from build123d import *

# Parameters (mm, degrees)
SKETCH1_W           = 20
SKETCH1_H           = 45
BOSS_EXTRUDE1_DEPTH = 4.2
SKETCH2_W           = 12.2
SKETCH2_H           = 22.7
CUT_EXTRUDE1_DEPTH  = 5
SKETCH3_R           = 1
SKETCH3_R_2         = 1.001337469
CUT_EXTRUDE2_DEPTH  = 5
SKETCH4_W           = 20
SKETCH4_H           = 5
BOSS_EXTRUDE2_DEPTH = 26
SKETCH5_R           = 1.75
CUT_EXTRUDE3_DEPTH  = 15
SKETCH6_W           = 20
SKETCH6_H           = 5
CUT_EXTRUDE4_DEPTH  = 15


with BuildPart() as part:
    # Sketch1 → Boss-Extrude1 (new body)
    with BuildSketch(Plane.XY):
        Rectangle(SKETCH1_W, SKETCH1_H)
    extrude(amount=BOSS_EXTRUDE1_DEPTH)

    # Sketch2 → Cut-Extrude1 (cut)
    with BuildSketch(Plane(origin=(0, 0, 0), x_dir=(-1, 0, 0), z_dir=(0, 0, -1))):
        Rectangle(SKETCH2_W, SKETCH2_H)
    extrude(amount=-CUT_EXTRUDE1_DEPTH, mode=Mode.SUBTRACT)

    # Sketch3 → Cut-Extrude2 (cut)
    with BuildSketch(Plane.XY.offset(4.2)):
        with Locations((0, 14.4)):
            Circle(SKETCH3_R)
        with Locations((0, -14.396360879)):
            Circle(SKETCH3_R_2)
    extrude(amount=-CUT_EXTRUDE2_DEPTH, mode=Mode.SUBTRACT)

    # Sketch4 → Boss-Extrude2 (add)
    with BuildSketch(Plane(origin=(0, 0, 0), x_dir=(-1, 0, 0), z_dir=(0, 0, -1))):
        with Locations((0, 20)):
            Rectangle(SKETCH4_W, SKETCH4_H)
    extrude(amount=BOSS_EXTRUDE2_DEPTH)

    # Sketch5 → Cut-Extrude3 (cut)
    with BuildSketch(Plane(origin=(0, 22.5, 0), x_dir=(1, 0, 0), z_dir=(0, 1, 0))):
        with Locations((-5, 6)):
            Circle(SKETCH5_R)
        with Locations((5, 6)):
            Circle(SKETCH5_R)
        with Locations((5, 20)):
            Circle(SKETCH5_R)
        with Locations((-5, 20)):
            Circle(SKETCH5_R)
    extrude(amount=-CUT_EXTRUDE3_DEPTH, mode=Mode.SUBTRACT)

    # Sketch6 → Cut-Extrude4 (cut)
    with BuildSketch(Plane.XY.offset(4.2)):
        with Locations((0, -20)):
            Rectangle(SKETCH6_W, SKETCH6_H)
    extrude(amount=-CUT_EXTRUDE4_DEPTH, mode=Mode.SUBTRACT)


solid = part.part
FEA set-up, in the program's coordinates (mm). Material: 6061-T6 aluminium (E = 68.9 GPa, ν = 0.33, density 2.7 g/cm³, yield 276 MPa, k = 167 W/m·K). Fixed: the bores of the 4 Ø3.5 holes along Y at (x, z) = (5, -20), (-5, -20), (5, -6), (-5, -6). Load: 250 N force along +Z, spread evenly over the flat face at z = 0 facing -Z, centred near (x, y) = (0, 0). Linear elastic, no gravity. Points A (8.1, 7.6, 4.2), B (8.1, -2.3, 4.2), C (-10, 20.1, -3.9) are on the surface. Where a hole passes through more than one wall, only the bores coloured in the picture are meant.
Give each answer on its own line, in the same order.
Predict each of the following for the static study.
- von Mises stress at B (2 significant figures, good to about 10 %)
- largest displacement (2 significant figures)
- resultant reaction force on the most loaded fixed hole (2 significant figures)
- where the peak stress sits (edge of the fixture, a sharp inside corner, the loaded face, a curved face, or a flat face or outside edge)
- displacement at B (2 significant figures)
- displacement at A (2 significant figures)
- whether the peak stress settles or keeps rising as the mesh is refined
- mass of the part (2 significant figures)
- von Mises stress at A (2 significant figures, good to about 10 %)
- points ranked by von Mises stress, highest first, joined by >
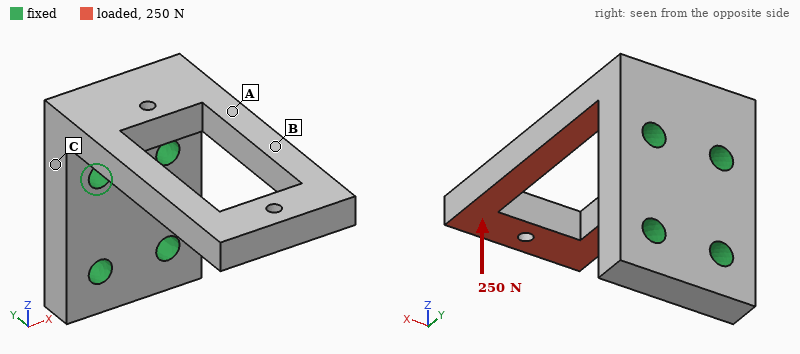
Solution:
46 MPa
0.47 mm
130 N
a sharp inside corner
0.21 mm
0.079 mm
keeps rising
12 g
100 MPa
A > B > C
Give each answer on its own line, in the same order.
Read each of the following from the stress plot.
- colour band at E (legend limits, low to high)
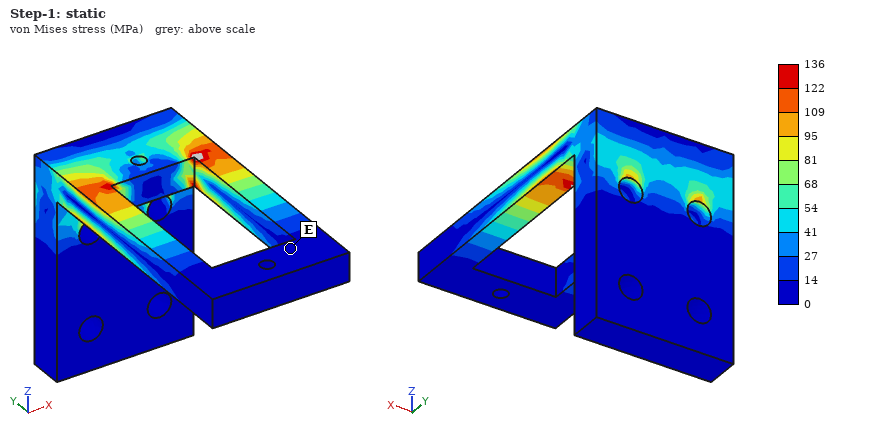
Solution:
0 to 14 MPa
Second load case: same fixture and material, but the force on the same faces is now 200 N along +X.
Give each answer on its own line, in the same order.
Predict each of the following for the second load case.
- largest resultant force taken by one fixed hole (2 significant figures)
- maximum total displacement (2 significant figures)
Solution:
300 N
0.11 mm
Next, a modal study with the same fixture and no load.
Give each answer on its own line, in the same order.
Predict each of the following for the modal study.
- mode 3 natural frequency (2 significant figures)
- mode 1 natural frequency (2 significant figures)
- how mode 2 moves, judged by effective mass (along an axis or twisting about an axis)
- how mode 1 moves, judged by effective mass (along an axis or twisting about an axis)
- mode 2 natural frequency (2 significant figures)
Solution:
5800 Hz
2000 Hz
along X
along Z
3700 Hz
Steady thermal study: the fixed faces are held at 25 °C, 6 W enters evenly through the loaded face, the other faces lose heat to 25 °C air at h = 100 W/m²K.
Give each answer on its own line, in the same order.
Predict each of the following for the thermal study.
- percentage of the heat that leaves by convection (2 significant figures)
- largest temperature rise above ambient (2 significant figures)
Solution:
20 %
15 K
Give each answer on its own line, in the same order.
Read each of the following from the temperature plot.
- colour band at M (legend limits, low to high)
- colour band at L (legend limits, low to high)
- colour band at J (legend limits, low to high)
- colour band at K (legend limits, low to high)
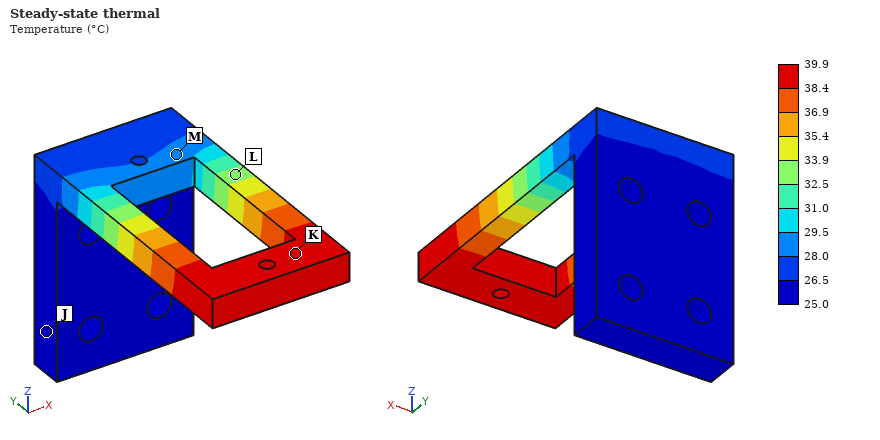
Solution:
28.0 to 29.5 °C
32.5 to 33.9 °C
25.0 to 26.5 °C
38.4 to 39.9 °C
